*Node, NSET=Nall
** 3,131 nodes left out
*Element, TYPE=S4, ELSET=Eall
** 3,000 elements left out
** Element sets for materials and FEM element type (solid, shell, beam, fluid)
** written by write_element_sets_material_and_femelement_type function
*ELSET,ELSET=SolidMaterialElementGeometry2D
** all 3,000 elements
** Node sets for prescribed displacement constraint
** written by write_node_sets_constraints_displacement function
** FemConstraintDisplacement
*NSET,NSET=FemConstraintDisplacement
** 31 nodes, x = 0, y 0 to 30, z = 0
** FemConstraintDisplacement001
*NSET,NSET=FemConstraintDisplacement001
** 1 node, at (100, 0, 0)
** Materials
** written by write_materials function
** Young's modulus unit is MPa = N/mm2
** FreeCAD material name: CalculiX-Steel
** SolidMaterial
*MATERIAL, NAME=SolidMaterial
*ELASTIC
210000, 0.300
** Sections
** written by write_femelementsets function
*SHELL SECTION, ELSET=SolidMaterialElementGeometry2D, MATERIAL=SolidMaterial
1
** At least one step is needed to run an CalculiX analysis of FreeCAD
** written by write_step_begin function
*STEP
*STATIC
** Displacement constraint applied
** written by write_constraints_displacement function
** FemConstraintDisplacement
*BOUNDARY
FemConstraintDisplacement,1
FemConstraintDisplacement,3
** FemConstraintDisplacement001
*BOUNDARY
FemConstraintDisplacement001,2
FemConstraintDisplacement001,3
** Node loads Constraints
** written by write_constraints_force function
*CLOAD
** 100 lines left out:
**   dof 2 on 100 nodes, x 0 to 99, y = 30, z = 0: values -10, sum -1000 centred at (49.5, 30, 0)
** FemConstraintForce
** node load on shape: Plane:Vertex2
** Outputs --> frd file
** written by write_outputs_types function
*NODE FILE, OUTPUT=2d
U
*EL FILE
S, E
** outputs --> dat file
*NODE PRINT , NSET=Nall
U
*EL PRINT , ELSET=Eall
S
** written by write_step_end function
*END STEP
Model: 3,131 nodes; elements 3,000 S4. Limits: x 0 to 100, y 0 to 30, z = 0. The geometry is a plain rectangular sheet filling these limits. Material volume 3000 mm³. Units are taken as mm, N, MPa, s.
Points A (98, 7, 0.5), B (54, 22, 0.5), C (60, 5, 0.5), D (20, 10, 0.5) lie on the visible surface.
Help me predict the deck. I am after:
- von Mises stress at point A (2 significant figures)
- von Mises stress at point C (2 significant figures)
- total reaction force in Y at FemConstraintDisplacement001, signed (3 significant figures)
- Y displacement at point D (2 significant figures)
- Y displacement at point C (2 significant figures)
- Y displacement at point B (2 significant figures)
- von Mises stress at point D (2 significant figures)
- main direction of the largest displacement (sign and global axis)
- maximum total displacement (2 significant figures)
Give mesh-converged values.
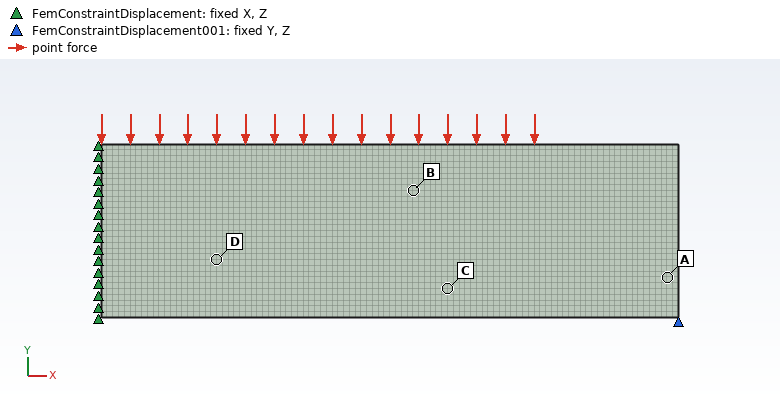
230 MPa
150 MPa
1000 N
-0.49 mm
-0.33 mm
-0.36 mm
110 MPa
-Y
0.52 mm
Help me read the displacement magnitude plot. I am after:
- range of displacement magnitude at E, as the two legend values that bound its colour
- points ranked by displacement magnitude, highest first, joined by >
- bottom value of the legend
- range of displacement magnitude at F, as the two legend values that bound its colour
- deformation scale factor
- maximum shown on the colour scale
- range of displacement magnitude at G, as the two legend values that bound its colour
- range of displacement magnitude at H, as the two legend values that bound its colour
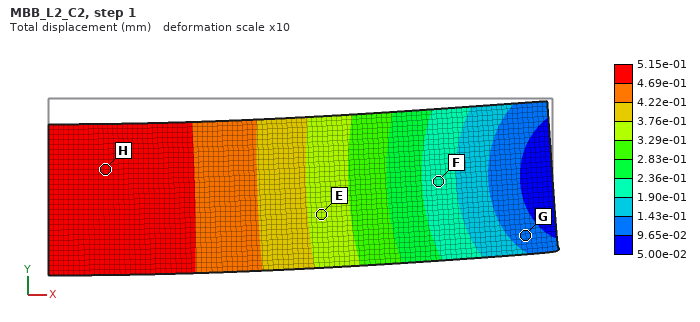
3.29e-01 to 3.76e-01 mm
H > E > F > G
5.00e-02 mm
1.90e-01 to 2.36e-01 mm
10
5.15e-01 mm
9.65e-02 to 1.43e-01 mm
4.69e-01 to 5.15e-01 mm
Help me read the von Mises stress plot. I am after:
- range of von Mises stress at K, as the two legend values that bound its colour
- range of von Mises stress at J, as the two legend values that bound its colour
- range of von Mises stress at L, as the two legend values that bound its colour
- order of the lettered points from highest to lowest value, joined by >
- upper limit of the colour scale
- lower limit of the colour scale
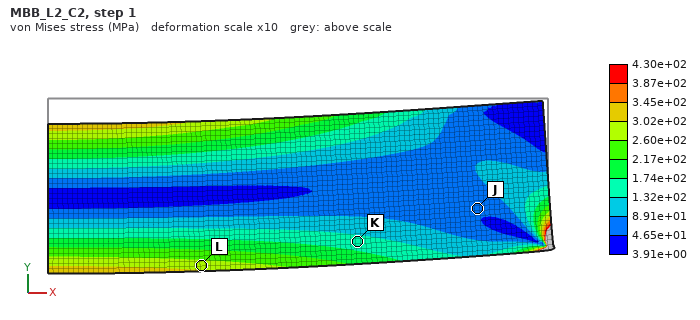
1.32e+02 to 1.74e+02 MPa
4.65e+01 to 8.91e+01 MPa
2.60e+02 to 3.02e+02 MPa
L > K > J
4.30e+02 MPa
3.91e+00 MPa
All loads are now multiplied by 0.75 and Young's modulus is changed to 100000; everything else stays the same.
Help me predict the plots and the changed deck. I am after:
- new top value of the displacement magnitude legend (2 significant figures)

0.81 mm
